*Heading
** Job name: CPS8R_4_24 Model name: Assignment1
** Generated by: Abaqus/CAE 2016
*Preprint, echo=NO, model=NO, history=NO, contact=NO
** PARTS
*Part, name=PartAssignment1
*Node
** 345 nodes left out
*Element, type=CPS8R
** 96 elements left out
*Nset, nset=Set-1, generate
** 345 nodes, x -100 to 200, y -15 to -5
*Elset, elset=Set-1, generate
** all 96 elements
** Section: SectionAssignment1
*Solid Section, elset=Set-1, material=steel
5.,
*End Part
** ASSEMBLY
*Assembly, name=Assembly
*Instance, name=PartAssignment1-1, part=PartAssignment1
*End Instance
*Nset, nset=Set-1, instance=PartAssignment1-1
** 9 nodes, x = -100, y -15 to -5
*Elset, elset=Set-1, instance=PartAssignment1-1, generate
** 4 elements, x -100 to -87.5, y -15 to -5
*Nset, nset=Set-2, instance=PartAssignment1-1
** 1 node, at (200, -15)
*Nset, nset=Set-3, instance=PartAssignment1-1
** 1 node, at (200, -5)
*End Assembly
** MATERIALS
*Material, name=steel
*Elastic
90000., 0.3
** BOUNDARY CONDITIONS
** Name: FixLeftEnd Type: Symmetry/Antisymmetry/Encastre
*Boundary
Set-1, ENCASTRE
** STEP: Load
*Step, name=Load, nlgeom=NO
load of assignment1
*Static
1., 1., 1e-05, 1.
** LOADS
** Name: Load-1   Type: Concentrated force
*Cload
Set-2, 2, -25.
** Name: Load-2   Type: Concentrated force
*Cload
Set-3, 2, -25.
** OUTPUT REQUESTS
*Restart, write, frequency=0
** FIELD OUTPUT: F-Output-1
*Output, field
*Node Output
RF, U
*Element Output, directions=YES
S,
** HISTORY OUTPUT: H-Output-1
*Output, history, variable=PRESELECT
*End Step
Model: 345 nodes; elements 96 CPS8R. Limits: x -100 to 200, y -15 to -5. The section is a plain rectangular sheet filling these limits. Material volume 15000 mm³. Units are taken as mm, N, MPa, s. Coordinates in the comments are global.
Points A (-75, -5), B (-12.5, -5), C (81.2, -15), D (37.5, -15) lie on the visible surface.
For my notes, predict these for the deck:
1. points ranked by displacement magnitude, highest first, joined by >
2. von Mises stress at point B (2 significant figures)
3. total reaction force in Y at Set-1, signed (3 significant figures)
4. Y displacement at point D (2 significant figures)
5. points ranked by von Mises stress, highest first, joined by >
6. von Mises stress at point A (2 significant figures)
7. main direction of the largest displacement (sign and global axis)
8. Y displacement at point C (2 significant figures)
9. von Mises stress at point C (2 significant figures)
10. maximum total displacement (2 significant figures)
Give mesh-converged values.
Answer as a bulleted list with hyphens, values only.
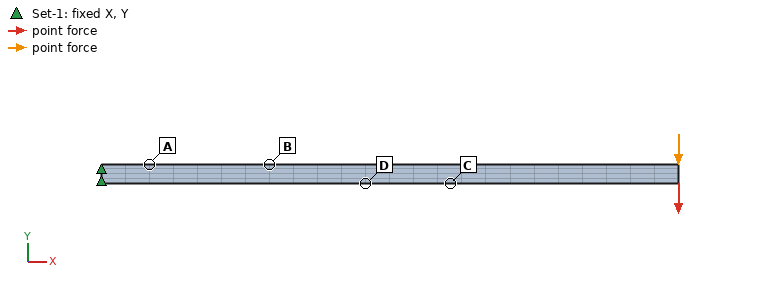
- C > D > B > A
- 130 MPa
- 50.0 N
- -3.2 mm
- A > B > D > C
- 160 MPa
- -Y
- -5.2 mm
- 70 MPa
- 12 mm
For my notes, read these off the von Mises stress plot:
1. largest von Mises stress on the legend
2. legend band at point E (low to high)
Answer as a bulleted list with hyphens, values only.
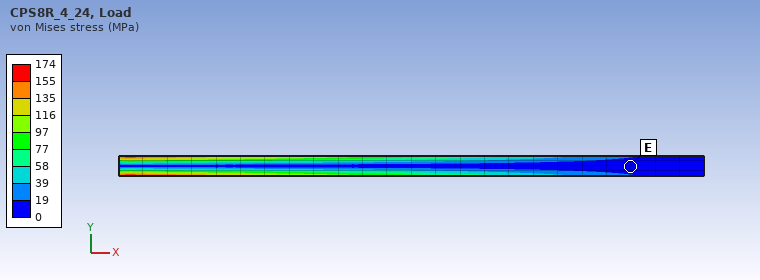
- 174 MPa
- 0 to 19 MPa
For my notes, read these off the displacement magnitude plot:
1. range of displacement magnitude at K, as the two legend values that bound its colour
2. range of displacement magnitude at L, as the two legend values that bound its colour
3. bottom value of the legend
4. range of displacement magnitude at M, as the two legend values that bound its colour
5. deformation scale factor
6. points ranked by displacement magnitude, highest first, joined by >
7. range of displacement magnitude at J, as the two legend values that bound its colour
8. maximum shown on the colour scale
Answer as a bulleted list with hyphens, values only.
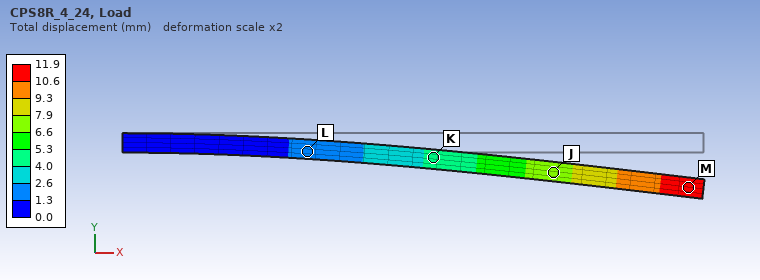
- 4.0 to 5.3 mm
- 1.3 to 2.6 mm
- 0.0 mm
- 10.6 to 11.9 mm
- 2
- M > J > K > L
- 6.6 to 7.9 mm
- 11.9 mm
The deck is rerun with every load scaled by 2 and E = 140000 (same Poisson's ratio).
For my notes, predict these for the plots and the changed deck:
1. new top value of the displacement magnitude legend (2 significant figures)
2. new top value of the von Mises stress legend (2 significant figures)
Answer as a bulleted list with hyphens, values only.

- 15 mm
- 350 MPa
